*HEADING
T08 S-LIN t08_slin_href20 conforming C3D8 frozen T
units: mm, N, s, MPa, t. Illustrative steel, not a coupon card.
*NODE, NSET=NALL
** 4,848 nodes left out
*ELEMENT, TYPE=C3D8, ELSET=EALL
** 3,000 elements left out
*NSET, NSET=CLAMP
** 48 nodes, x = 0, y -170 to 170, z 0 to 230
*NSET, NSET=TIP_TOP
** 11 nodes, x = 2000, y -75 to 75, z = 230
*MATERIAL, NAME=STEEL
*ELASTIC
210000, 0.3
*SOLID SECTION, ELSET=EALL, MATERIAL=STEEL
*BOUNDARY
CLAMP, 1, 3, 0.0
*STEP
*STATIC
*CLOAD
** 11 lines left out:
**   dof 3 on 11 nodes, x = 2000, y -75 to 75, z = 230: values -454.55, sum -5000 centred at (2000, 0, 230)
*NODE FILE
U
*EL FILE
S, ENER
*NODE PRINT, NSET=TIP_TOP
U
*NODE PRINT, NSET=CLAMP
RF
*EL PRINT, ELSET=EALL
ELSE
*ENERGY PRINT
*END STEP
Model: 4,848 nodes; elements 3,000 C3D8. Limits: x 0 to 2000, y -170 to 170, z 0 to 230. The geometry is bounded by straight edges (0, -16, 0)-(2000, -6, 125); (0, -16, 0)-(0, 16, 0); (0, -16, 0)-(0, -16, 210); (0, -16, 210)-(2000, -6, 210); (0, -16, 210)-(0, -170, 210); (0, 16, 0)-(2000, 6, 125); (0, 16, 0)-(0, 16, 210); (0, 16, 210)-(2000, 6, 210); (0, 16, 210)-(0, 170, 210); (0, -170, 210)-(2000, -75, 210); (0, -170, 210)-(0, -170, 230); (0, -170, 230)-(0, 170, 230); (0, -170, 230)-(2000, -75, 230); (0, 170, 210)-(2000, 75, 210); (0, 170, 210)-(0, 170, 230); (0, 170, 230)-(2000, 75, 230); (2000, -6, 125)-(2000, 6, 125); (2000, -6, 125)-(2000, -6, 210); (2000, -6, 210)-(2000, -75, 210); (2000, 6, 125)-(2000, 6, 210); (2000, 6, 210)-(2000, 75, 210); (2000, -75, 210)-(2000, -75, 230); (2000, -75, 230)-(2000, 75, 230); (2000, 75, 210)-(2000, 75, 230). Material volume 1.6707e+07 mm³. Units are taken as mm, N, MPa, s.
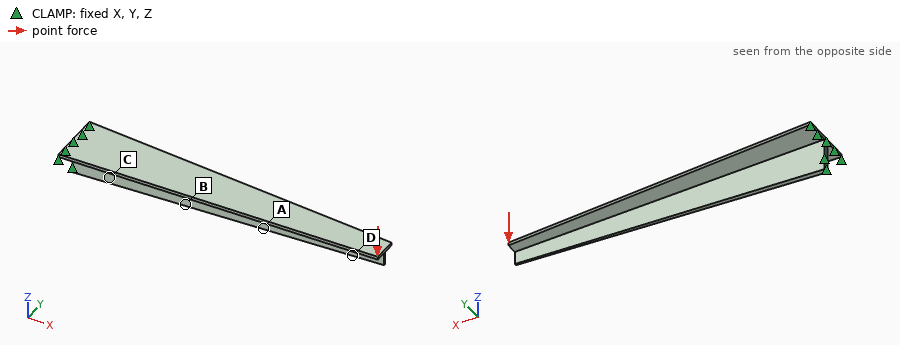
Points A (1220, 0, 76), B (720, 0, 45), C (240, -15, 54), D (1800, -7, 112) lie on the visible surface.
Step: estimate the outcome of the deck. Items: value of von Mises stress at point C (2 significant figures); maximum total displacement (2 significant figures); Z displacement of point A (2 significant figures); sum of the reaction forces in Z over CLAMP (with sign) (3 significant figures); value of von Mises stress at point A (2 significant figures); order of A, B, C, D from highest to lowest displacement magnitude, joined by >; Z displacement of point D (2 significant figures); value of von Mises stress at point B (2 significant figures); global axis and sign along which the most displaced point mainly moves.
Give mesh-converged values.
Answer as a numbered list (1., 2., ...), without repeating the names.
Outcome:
1. 19 MPa
2. 2.1 mm
3. -0.67 mm
4. 5000 N
5. 32 MPa
6. D > A > B > C
7. -1.6 mm
8. 30 MPa
9. -Z
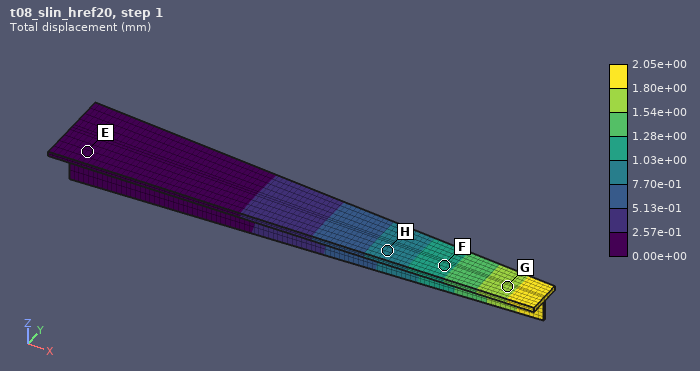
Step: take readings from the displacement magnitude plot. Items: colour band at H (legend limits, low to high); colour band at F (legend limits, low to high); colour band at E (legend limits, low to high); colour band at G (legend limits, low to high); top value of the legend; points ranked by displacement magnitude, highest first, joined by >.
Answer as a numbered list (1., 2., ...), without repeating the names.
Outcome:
1. 7.70e-01 to 1.03e+00 mm
2. 1.03e+00 to 1.28e+00 mm
3. 0.00e+00 to 2.57e-01 mm
4. 1.54e+00 to 1.80e+00 mm
5. 2.05e+00 mm
6. G > F > H > E
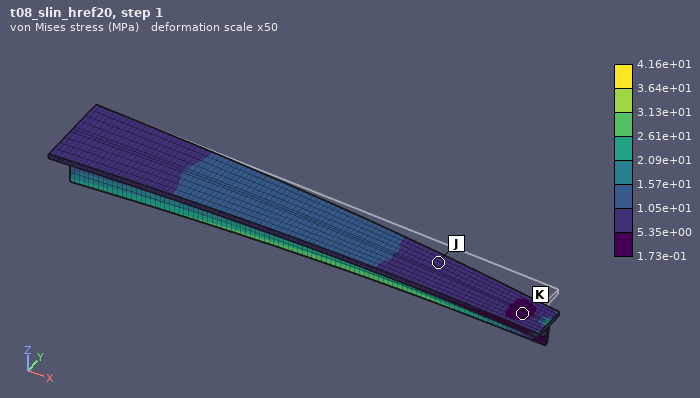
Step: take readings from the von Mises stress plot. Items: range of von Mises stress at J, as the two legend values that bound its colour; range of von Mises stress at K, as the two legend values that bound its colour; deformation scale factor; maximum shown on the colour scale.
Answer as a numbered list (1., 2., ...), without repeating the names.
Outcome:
1. 5.35e+00 to 1.05e+01 MPa
2. 1.73e-01 to 5.35e+00 MPa
3. 50
4. 4.16e+01 MPa
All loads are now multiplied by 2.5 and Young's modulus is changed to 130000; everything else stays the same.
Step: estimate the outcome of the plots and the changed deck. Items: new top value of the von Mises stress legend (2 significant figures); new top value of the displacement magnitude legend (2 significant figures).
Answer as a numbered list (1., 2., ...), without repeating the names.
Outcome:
1. 100 MPa
2. 8.3 mm
